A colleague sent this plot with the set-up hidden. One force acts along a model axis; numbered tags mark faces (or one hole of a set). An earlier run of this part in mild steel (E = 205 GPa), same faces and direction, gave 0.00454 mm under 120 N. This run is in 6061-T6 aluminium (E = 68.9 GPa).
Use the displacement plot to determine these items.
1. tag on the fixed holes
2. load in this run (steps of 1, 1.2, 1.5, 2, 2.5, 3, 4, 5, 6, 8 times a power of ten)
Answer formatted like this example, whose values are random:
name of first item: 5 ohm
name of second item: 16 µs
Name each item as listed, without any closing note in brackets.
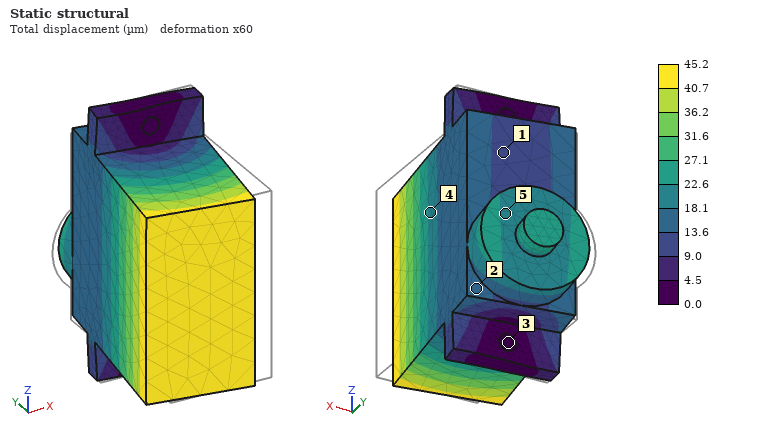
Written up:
tag on the fixed holes: 3
load in this run: 400 N
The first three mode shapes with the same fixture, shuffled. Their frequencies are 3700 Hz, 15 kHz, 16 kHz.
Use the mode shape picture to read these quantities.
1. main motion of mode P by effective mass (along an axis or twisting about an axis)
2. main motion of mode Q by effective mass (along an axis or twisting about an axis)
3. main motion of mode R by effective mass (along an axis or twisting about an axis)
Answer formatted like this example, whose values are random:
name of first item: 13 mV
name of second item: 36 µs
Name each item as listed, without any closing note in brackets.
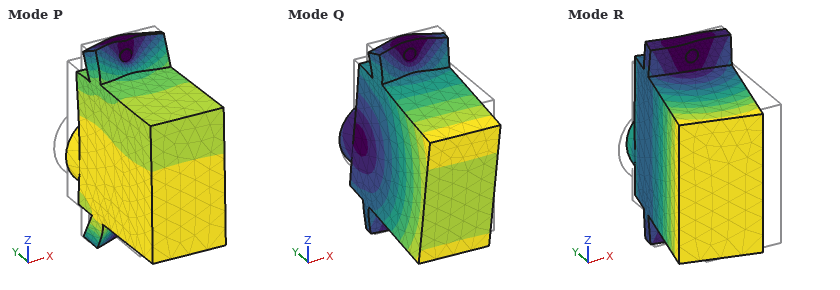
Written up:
main motion of mode P by effective mass: along Y
main motion of mode Q by effective mass: along Z
main motion of mode R by effective mass: along X
